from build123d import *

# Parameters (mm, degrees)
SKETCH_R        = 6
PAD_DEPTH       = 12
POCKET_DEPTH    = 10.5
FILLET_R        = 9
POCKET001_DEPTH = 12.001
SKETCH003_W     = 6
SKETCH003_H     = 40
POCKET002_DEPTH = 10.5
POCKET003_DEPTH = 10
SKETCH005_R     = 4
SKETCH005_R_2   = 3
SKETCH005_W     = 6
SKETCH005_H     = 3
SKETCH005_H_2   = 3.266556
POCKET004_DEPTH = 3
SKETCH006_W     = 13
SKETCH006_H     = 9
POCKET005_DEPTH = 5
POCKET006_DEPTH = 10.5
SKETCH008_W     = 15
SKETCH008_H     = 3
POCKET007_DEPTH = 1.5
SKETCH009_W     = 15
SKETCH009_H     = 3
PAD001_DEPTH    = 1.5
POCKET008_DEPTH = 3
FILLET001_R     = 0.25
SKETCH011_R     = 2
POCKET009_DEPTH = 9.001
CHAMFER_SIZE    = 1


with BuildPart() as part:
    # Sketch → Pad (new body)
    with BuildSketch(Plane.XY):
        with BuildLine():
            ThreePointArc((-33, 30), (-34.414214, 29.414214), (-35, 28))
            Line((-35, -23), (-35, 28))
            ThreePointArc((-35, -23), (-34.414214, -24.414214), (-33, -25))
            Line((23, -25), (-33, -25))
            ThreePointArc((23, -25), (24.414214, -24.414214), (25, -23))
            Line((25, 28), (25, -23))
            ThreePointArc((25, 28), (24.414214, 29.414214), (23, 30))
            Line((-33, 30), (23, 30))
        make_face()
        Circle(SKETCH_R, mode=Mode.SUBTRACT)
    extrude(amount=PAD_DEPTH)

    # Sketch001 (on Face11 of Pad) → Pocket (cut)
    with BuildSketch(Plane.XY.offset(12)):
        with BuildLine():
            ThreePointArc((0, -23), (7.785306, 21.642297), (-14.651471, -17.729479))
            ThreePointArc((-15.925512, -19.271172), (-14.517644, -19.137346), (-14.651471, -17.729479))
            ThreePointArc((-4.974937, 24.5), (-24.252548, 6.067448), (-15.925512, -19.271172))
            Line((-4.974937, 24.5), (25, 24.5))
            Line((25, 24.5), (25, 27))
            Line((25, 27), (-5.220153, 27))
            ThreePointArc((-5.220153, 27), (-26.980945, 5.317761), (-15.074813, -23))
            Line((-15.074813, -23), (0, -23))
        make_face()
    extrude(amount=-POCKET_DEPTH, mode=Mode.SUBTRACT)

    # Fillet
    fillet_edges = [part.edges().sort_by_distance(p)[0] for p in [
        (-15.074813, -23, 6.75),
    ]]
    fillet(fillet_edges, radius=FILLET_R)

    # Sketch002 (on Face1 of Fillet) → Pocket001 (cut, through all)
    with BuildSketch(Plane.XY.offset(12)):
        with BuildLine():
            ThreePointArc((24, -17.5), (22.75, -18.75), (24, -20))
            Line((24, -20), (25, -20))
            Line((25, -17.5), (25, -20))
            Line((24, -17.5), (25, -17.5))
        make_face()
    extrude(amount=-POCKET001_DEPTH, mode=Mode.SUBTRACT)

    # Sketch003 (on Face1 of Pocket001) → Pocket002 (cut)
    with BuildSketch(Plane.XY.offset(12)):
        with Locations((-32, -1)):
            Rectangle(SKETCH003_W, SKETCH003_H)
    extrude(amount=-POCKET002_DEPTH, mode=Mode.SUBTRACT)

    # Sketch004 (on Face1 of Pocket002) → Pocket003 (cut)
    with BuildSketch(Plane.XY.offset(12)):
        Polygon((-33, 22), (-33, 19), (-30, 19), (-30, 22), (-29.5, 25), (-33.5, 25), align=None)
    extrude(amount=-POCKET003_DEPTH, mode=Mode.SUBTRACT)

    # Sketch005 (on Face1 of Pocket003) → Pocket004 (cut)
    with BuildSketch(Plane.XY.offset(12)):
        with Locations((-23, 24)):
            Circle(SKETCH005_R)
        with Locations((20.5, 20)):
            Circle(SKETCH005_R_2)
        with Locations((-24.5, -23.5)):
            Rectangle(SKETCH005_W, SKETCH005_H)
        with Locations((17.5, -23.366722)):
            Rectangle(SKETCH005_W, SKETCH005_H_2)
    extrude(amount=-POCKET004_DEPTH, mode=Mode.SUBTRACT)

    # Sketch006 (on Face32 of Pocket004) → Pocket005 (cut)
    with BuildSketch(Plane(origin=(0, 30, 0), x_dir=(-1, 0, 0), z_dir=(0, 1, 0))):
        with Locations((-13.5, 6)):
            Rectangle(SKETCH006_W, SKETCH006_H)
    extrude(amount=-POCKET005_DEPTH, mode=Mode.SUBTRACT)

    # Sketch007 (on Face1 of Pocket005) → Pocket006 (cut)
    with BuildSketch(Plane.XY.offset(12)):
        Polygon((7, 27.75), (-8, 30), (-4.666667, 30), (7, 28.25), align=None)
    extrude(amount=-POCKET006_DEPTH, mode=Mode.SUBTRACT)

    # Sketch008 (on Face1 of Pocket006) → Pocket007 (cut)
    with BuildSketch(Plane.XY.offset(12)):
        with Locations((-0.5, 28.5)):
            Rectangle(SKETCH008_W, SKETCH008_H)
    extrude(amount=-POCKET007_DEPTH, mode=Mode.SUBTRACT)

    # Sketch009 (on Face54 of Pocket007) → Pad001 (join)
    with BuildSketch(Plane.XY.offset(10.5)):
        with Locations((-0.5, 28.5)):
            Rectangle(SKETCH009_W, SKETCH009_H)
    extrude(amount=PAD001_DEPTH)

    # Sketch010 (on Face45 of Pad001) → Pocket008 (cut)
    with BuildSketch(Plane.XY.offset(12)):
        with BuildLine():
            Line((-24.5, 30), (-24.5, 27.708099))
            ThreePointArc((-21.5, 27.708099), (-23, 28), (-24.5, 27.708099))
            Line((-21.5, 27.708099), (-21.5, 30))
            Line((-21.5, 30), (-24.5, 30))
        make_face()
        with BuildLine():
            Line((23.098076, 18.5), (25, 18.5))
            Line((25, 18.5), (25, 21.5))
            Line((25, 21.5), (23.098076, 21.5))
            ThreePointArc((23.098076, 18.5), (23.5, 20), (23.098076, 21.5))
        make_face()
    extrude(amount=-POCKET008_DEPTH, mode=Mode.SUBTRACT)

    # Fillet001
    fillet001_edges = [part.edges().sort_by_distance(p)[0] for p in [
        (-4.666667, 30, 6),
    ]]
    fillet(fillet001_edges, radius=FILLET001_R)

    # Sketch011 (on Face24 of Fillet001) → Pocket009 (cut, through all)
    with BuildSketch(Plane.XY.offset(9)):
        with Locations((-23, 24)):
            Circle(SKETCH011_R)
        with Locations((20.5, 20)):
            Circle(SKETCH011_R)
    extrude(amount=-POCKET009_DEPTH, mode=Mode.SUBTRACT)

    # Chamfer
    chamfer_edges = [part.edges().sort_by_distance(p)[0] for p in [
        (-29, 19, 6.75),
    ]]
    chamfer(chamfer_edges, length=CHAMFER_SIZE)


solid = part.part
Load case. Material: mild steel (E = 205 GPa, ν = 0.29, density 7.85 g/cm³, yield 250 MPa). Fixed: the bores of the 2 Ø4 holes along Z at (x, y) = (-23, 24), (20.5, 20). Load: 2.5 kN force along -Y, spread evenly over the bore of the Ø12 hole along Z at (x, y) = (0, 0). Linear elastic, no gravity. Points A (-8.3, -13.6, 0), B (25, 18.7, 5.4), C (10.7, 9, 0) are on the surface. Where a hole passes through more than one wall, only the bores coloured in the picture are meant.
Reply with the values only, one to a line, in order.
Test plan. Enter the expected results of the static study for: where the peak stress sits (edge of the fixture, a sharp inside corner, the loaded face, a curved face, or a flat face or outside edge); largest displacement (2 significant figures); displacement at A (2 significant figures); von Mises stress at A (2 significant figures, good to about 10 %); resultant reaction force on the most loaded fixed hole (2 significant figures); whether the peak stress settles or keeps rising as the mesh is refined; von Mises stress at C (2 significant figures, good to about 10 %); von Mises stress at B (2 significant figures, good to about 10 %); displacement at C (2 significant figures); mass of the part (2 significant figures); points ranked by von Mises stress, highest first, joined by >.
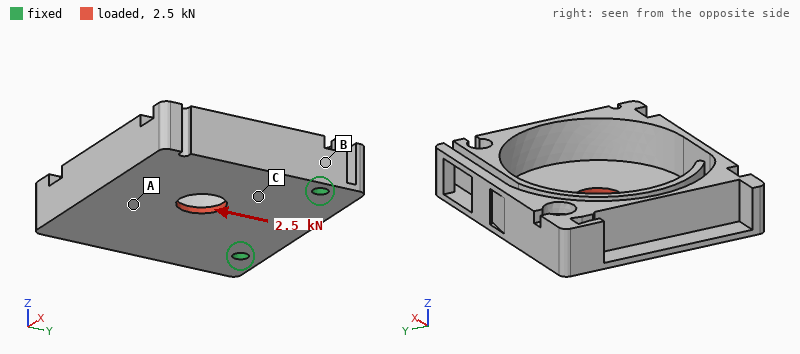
edge of the fixture
14 µm
7.9 µm
22 MPa
1.3 kN
keeps rising
39 MPa
10 MPa
4.2 µm
120 g
C > A > B
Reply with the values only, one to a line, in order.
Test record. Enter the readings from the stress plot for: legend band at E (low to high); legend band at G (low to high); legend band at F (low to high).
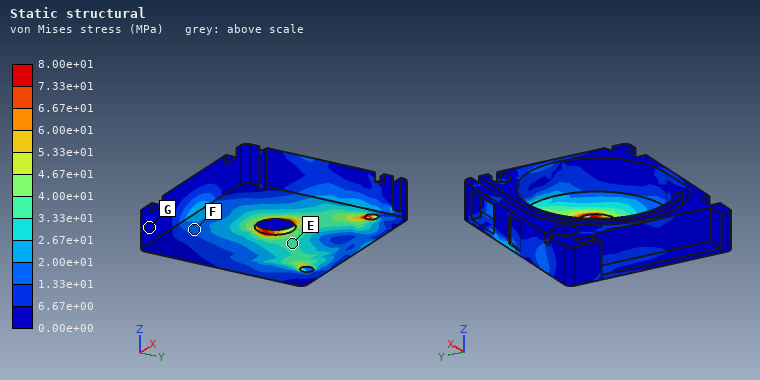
3.33e+01 to 4.00e+01 MPa
0.00e+00 to 6.67e+00 MPa
1.33e+01 to 2.00e+01 MPa
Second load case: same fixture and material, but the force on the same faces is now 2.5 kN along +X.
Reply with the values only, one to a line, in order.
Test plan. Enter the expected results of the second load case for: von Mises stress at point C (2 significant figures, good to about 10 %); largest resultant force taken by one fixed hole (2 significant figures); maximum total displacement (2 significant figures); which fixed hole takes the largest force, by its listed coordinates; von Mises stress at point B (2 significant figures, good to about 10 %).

54 MPa
1.8 kN
17 µm
(20.5, 20)
32 MPa
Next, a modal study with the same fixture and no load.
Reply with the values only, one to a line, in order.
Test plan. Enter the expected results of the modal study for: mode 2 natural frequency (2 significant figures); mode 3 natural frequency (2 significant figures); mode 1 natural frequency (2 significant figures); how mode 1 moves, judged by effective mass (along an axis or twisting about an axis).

3400 Hz
6600 Hz
2400 Hz
along Z
